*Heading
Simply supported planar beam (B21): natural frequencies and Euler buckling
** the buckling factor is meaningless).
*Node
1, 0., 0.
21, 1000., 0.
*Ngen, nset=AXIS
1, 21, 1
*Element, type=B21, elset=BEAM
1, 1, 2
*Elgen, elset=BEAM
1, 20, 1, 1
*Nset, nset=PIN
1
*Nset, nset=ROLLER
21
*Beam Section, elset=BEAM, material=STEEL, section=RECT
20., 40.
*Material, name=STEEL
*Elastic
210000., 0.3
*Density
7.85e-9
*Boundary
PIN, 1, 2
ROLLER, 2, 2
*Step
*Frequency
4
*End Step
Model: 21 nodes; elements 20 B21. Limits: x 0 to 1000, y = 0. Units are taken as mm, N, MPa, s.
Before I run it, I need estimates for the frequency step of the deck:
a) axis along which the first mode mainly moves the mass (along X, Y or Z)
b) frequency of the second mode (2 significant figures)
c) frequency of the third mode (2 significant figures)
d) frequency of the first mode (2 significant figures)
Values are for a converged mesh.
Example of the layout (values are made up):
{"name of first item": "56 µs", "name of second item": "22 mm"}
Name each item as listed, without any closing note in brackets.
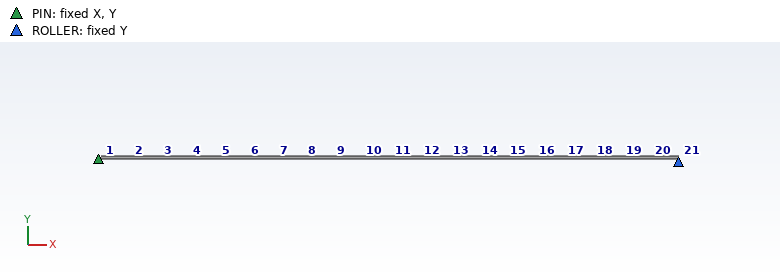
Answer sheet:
{"axis along which the first mode mainly moves the mass": "along Y", "frequency of the second mode": "370 Hz", "frequency of the third mode": "820 Hz", "frequency of the first mode": "94 Hz"}
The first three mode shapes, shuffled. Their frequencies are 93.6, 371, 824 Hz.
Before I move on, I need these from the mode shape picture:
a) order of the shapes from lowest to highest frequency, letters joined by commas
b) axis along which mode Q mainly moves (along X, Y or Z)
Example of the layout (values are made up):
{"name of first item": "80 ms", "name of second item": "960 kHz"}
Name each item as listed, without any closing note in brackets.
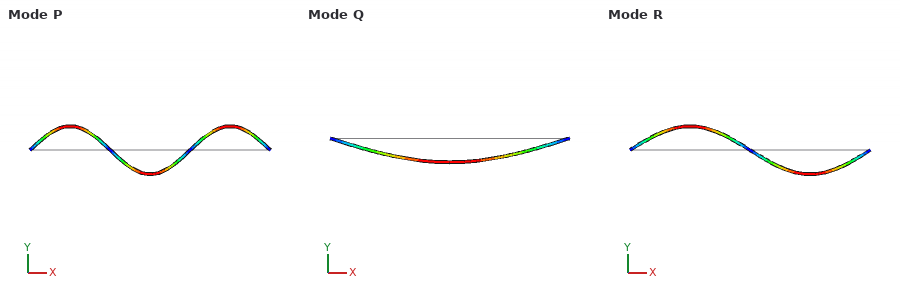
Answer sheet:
{"order of the shapes from lowest to highest frequency, letters joined by commas": "Q, R, P", "axis along which mode Q mainly moves": "along Y"}
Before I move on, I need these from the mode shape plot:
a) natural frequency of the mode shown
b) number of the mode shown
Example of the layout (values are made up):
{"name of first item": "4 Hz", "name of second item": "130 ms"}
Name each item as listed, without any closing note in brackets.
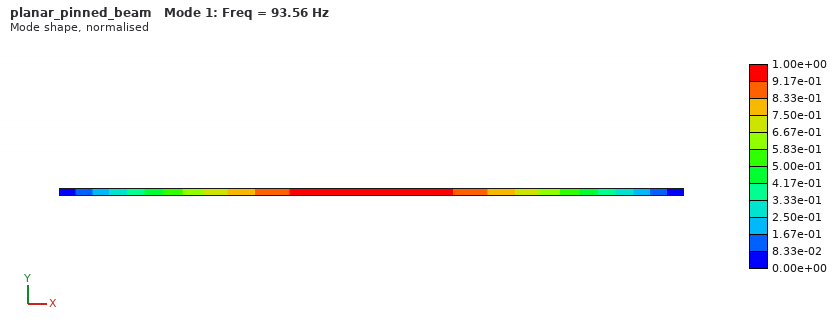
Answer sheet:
{"natural frequency of the mode shown": "93.56 Hz", "number of the mode shown": "1"}
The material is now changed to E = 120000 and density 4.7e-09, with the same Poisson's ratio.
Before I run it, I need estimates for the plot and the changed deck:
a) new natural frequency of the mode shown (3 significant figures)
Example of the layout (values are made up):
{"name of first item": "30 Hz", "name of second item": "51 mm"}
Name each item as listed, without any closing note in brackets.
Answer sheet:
{"new natural frequency of the mode shown": "91.4 Hz"}
